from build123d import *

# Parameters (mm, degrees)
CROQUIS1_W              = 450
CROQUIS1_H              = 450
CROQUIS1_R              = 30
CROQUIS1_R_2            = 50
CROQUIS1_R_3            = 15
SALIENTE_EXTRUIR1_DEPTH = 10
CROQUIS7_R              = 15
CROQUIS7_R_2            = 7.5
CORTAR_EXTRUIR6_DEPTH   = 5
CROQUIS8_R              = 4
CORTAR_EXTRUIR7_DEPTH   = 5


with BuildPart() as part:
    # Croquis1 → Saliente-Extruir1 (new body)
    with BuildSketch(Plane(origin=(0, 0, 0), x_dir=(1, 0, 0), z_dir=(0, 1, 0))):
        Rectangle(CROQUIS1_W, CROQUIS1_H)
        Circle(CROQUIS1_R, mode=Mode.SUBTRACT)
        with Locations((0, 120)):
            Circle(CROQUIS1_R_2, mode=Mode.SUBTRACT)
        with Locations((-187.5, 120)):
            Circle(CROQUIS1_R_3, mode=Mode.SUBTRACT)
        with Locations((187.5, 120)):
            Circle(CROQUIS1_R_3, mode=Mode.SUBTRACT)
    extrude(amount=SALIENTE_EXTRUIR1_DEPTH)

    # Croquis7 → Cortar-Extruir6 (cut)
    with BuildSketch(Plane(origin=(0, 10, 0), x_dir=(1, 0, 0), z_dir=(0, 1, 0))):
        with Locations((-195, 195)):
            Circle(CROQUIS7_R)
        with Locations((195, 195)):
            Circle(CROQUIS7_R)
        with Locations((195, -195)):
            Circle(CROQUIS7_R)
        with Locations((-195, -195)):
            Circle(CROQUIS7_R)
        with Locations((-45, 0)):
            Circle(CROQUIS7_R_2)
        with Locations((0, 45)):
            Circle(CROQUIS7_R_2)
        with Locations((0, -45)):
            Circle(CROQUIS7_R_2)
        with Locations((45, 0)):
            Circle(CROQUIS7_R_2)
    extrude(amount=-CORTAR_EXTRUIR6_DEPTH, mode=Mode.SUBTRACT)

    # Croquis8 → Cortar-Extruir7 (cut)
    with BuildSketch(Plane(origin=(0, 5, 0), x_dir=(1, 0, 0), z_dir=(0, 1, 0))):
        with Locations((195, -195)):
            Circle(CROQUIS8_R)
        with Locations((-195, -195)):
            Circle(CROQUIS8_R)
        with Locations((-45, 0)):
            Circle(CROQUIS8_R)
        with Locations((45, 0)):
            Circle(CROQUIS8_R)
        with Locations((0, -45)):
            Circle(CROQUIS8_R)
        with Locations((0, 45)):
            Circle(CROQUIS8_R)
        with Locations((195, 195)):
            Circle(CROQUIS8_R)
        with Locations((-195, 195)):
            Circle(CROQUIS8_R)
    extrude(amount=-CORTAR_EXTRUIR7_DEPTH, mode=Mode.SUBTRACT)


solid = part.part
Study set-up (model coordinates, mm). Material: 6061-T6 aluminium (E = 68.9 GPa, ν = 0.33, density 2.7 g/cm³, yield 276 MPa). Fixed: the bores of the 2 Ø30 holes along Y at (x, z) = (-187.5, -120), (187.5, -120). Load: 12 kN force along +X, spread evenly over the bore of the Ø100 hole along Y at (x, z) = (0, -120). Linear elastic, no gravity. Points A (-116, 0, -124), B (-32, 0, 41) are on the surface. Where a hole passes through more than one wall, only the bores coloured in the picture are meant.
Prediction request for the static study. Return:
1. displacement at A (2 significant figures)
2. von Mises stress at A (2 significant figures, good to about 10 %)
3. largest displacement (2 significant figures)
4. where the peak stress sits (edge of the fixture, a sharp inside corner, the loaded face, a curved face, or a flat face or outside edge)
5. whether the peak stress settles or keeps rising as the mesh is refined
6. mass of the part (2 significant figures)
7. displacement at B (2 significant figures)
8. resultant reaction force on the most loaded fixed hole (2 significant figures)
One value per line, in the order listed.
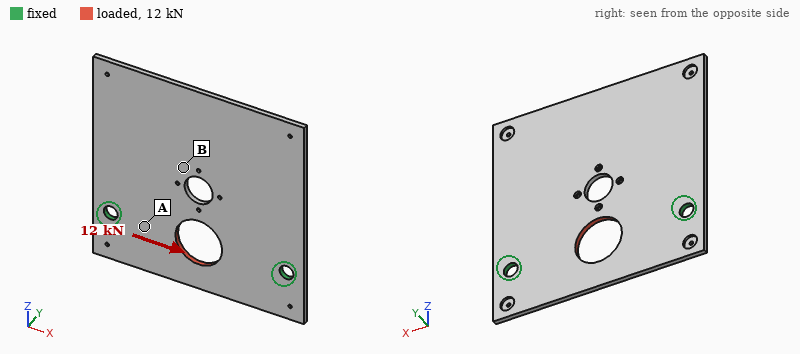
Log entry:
6.0 µm
5.6 MPa
13 µm
edge of the fixture
keeps rising
5.1 kg
7.5 µm
6.0 kN
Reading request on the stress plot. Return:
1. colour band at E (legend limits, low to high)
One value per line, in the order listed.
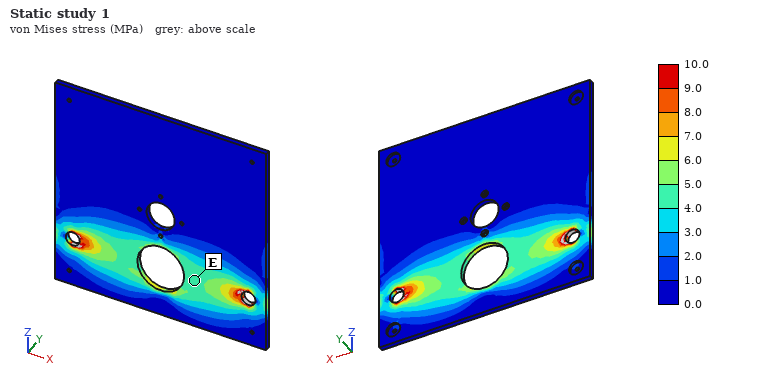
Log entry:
4.0 to 5.0 MPa
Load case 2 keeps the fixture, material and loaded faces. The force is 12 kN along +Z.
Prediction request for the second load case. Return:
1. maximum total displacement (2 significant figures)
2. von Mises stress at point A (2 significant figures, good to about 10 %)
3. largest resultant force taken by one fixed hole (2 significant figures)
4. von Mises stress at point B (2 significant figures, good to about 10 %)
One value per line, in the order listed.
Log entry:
29 µm
3.9 MPa
6.0 kN
3.2 MPa
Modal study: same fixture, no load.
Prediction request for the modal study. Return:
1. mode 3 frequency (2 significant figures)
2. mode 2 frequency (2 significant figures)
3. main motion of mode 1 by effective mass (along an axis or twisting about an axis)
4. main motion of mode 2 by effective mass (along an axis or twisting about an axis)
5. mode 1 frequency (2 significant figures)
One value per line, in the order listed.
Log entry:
320 Hz
140 Hz
along Y
twisting about Z
61 Hz
